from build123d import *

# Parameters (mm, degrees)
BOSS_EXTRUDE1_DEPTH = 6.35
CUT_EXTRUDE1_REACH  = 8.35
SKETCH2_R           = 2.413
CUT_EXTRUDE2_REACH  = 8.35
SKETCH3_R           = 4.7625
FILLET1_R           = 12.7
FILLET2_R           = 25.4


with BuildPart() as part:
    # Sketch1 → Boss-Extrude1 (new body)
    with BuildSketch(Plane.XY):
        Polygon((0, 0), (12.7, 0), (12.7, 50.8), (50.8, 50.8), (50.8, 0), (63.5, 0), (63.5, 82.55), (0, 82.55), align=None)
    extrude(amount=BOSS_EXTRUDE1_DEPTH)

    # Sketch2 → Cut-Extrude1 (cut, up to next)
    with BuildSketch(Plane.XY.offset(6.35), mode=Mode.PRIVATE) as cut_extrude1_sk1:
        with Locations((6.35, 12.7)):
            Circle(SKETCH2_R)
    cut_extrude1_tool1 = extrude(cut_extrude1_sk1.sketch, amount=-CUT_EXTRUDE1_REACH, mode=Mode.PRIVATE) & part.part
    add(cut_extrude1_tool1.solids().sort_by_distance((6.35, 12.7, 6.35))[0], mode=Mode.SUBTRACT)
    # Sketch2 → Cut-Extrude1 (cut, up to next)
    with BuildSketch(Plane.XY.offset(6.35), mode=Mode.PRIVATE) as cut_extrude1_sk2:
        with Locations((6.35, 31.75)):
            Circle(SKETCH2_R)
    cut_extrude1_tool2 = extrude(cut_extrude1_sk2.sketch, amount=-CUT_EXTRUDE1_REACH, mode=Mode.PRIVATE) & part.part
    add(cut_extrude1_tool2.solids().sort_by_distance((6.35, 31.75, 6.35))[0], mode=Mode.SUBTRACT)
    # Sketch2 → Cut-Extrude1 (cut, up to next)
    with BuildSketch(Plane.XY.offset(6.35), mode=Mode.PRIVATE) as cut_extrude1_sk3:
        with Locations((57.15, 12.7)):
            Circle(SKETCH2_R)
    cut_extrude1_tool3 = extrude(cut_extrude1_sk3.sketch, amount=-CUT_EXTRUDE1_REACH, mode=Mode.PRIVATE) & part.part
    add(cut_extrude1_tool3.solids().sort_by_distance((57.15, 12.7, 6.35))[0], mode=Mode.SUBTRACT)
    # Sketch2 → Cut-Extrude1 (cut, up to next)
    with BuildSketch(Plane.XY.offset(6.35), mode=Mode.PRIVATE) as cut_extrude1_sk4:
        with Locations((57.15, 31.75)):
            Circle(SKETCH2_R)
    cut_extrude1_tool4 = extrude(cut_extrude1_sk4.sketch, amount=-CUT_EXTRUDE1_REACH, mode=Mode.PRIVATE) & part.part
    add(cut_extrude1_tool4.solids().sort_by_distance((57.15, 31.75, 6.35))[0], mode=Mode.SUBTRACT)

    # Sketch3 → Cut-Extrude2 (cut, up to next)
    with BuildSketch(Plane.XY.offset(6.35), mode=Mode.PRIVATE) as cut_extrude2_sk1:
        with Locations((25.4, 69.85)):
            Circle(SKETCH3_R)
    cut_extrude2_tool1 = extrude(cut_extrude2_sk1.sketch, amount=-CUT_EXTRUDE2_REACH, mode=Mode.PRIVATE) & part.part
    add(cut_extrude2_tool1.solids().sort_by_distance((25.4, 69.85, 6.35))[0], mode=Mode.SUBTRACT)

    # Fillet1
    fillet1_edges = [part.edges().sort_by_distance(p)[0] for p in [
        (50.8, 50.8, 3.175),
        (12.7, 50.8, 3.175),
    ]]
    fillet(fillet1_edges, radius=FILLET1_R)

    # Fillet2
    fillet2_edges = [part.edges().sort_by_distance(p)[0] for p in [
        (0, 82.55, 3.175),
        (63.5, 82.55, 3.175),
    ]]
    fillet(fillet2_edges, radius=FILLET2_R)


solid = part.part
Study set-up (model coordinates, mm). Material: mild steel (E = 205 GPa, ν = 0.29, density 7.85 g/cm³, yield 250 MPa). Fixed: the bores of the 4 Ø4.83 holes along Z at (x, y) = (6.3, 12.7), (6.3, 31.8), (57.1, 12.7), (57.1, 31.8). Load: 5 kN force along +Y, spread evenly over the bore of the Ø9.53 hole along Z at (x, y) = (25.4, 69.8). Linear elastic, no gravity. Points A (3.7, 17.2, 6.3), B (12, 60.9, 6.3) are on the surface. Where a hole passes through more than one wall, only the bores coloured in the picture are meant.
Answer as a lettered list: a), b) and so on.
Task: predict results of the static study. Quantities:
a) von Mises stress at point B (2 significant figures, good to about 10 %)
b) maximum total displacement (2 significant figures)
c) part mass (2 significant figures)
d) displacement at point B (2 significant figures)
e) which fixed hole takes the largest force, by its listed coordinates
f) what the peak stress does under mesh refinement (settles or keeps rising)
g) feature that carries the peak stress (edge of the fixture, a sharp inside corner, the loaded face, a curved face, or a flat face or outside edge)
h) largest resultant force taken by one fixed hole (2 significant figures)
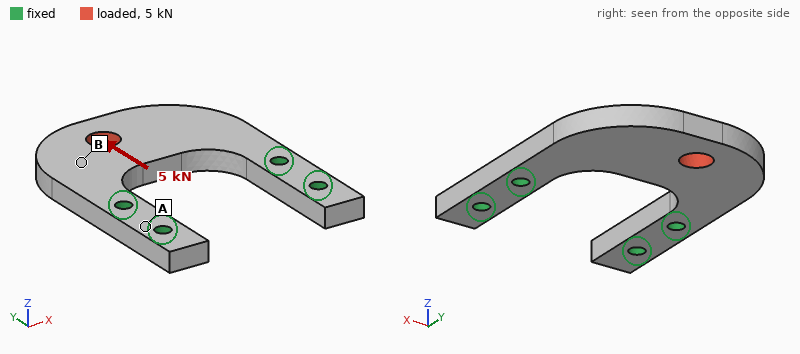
a) 30 MPa
b) 9.3 µm
c) 150 g
d) 5.2 µm
e) (6.3, 31.8)
f) keeps rising
g) edge of the fixture
h) 3.1 kN
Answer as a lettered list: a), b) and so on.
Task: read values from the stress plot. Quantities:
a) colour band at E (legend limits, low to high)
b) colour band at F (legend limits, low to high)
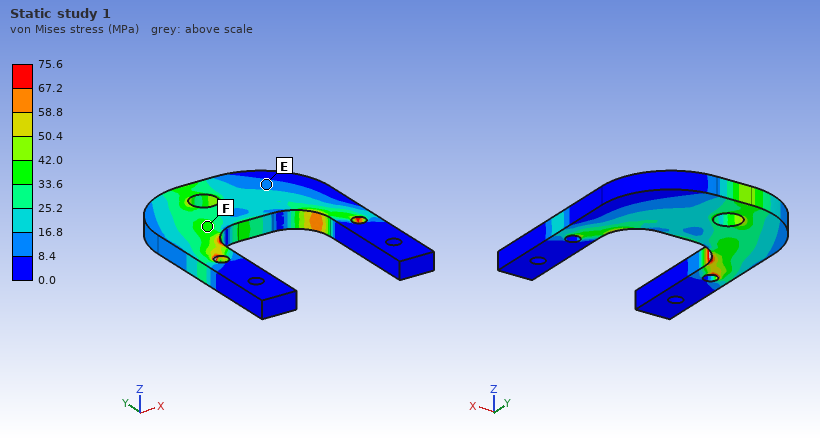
a) 8.4 to 16.8 MPa
b) 33.6 to 42.0 MPa
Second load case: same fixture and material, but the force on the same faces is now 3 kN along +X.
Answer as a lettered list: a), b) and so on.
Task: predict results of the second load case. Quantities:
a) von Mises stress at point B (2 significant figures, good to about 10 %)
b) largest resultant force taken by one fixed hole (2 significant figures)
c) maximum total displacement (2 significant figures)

a) 12 MPa
b) 2.4 kN
c) 16 µm
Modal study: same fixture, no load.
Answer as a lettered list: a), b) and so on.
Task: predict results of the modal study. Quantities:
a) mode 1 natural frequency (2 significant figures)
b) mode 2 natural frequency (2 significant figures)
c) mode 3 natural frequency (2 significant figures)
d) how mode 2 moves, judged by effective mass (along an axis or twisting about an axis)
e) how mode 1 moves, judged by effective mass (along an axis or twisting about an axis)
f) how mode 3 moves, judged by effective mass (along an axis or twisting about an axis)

a) 1600 Hz
b) 4700 Hz
c) 8100 Hz
d) twisting about Y
e) along Z
f) along X
